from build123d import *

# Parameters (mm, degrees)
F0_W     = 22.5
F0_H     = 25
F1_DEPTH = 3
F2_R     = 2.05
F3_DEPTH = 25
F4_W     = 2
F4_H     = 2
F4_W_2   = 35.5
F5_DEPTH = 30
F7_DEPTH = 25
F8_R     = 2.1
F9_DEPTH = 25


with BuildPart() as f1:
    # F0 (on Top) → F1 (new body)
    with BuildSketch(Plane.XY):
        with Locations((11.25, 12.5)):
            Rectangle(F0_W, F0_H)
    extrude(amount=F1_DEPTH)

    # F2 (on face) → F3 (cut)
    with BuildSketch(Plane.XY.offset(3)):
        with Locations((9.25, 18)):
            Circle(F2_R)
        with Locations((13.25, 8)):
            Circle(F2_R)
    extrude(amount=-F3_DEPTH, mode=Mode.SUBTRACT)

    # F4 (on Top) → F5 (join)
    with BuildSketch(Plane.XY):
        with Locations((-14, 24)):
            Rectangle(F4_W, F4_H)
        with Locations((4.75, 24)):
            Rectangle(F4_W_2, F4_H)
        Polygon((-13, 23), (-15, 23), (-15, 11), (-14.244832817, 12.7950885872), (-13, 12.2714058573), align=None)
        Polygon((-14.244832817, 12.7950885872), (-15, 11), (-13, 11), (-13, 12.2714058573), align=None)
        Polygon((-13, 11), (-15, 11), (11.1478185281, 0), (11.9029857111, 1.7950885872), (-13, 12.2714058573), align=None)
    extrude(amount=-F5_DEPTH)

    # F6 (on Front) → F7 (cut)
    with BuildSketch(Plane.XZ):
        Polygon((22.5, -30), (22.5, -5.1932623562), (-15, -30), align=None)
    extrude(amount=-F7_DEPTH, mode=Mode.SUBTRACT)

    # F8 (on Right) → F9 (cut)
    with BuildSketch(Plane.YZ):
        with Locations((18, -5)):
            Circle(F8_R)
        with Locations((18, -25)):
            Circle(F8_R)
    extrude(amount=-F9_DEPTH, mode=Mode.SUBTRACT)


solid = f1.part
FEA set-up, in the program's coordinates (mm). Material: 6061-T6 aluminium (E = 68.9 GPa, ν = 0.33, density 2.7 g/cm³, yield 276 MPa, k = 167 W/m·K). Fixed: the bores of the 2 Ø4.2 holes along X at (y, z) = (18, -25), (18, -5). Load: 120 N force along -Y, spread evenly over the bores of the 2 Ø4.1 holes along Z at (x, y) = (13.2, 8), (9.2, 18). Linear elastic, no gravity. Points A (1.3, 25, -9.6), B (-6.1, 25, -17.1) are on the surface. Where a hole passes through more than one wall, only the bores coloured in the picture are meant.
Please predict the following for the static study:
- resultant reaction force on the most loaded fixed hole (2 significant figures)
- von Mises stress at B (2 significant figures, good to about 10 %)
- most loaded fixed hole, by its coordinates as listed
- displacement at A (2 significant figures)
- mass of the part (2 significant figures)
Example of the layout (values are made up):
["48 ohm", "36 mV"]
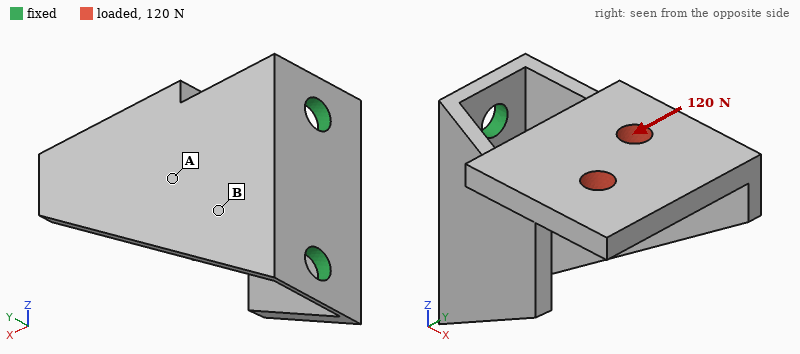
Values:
["140 N", "30 MPa", "(18, -5)", "0.12 mm", "13 g"]
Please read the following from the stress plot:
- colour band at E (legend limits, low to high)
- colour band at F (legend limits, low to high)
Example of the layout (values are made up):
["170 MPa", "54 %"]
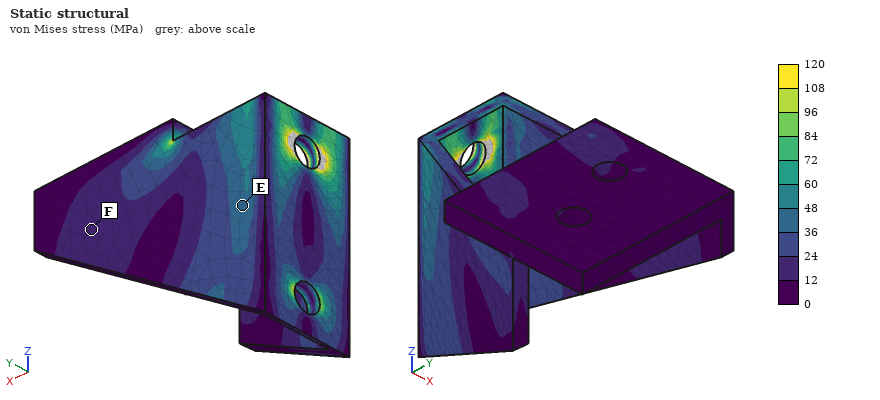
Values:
["36 to 48 MPa", "12 to 24 MPa"]
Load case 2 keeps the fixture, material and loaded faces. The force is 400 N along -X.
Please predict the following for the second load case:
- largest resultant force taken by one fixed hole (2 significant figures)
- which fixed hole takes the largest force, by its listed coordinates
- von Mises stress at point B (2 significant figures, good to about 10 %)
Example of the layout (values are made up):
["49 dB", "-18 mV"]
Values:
["510 N", "(18, -5)", "24 MPa"]
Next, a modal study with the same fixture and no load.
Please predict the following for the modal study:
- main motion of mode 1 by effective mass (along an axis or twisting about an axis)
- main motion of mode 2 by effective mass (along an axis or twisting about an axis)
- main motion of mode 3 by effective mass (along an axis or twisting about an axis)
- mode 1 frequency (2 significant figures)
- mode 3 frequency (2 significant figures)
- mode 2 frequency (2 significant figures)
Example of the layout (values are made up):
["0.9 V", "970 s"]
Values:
["along Y", "along Z", "along X", "1400 Hz", "6400 Hz", "4600 Hz"]
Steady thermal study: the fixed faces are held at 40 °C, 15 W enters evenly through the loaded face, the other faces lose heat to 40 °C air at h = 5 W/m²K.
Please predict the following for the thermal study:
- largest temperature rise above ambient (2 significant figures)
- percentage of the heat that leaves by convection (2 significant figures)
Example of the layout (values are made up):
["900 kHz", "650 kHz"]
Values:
["44 K", "3.3 %"]
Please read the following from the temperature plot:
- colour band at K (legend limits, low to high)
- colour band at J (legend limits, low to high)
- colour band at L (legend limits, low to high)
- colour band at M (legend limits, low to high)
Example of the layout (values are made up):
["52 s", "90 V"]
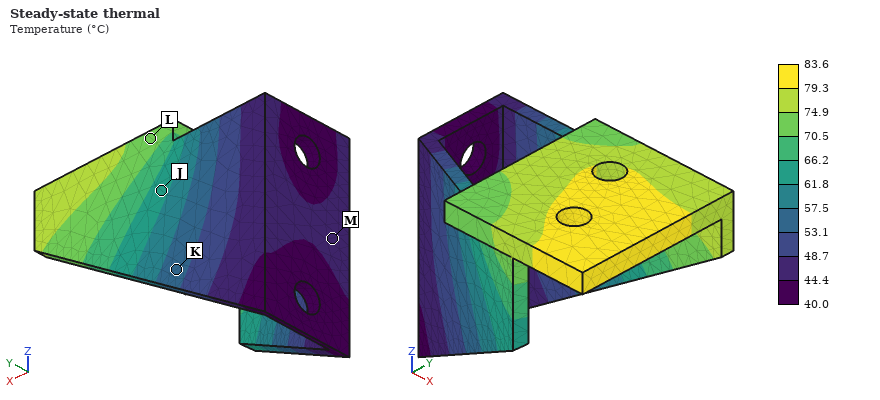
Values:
["53.1 to 57.5 °C", "61.8 to 66.2 °C", "70.5 to 74.9 °C", "44.4 to 48.7 °C"]
